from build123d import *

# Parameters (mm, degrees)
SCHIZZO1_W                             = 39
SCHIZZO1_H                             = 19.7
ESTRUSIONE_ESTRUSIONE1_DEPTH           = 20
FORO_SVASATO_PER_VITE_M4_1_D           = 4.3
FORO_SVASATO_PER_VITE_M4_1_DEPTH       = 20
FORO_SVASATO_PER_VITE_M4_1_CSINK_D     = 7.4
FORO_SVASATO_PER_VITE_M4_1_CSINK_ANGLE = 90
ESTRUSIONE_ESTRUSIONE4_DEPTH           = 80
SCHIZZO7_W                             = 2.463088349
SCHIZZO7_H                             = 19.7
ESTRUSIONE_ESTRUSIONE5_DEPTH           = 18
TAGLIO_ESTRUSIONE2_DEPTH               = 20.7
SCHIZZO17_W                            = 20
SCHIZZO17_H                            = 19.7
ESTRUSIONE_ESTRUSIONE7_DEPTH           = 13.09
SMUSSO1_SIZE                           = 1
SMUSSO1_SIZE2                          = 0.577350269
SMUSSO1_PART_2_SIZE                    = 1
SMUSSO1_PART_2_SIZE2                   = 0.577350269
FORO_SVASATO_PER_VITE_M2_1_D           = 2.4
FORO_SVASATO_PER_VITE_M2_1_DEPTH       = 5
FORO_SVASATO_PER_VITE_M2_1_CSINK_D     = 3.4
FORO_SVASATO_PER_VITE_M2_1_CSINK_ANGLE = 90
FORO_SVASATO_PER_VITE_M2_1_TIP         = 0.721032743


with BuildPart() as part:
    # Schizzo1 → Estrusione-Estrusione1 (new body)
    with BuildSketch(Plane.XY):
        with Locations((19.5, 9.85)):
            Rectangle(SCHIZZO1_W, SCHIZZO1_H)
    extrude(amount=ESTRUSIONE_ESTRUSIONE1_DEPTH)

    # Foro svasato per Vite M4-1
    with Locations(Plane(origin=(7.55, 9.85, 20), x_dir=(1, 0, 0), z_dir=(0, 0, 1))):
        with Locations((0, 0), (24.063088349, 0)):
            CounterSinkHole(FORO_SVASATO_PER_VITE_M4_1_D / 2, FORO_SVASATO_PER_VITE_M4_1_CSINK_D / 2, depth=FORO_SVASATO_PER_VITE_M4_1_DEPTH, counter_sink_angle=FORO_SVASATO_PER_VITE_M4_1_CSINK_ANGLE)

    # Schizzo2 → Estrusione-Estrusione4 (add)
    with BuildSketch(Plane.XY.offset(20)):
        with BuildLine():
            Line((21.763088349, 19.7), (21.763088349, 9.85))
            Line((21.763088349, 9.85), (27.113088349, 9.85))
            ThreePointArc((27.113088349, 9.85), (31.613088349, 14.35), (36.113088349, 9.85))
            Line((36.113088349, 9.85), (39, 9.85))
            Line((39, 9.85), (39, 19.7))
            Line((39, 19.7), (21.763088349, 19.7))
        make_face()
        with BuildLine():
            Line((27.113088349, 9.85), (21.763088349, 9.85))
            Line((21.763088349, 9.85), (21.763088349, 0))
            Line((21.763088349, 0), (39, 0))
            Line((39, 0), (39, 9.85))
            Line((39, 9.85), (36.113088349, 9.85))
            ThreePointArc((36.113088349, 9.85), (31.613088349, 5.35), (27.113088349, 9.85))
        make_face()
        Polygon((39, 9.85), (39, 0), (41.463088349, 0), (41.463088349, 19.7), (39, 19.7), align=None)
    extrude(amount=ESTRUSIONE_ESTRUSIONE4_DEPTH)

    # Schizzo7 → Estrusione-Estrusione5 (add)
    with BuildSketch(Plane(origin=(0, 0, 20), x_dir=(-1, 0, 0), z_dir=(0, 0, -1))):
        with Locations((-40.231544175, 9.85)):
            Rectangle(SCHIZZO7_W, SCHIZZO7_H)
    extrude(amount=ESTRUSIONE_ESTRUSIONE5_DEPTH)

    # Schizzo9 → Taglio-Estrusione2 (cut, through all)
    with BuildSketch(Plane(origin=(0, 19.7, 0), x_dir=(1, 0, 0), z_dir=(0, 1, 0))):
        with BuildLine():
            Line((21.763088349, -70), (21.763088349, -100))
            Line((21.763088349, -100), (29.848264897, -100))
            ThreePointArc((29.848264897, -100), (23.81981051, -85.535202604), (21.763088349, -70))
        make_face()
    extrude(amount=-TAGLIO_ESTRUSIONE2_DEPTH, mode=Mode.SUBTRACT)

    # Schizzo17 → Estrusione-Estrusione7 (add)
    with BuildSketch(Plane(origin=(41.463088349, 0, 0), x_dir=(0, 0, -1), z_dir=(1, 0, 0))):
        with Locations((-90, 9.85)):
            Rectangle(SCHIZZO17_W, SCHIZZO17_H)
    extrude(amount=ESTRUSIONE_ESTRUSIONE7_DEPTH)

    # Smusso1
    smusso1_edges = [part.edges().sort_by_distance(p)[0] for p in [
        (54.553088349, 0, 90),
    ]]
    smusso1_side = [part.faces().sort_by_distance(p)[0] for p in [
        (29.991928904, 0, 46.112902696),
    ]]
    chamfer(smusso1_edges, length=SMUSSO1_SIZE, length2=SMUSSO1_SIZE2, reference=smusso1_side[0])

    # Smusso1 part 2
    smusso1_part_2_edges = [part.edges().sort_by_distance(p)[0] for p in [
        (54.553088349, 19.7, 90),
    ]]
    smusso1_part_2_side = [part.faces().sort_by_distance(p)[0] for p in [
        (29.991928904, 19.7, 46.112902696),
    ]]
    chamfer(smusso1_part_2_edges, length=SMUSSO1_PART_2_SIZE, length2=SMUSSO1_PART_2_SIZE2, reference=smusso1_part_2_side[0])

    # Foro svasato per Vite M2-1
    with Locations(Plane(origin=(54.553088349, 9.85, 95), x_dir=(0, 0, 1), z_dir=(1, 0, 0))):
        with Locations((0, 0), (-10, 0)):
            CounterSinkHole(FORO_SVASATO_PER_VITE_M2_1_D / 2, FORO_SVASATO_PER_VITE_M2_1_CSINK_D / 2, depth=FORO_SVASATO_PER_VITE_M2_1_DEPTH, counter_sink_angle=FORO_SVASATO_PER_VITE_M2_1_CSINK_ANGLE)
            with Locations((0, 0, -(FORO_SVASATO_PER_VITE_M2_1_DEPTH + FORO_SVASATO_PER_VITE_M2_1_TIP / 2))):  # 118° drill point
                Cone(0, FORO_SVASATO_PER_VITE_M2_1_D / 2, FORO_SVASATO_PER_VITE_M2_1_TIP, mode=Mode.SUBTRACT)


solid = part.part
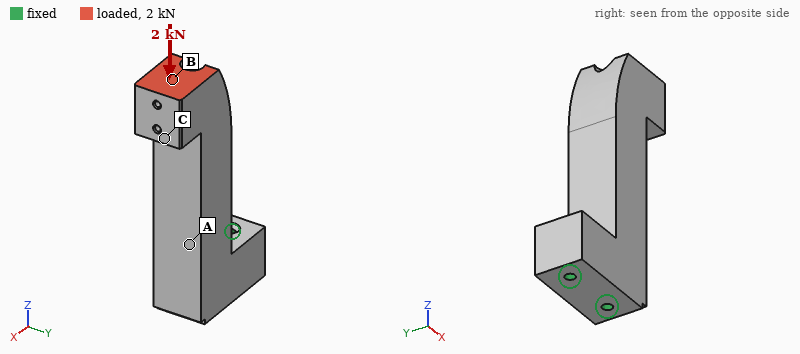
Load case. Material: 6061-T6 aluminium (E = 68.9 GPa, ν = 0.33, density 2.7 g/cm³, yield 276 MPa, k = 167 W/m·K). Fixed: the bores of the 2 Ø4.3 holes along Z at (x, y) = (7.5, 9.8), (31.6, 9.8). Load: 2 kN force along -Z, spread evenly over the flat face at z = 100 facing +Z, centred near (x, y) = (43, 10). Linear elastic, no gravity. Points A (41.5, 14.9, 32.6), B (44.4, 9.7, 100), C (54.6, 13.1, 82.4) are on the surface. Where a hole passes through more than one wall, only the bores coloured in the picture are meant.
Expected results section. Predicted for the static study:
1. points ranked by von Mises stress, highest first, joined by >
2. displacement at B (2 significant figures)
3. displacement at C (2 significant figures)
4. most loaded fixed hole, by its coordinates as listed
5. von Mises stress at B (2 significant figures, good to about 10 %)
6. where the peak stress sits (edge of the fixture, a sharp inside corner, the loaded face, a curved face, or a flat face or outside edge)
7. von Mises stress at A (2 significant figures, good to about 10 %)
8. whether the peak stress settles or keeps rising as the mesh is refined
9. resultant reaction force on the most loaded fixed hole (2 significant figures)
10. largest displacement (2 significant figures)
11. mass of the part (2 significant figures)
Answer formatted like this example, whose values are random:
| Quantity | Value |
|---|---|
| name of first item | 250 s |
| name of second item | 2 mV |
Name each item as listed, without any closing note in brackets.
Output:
| Quantity | Value |
|---|---|
| points ranked by von Mises stress, highest first, joined by > | A > B > C |
| displacement at B | 0.12 mm |
| displacement at C | 0.097 mm |
| most loaded fixed hole, by its coordinates as listed | (31.6, 9.8) |
| von Mises stress at B | 6.2 MPa |
| where the peak stress sits | edge of the fixture |
| von Mises stress at A | 25 MPa |
| whether the peak stress settles or keeps rising as the mesh is refined | keeps rising |
| resultant reaction force on the most loaded fixed hole | 2.4 kN |
| largest displacement | 0.13 mm |
| mass of the part | 120 g |
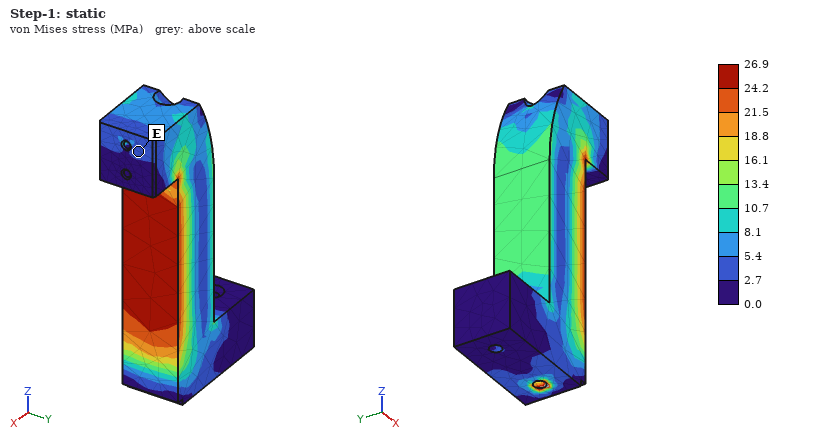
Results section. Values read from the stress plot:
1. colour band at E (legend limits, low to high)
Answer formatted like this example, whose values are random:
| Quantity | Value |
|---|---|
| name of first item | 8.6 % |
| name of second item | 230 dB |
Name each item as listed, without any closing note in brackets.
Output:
| Quantity | Value |
|---|---|
| colour band at E | 2.7 to 5.4 MPa |
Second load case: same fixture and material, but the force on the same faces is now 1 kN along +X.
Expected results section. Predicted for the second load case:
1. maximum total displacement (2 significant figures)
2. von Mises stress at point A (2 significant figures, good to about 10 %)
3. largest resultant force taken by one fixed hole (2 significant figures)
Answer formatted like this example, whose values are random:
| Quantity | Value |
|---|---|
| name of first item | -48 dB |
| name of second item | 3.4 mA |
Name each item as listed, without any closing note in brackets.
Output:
| Quantity | Value |
|---|---|
| maximum total displacement | 0.33 mm |
| von Mises stress at point A | 55 MPa |
| largest resultant force taken by one fixed hole | 2.5 kN |
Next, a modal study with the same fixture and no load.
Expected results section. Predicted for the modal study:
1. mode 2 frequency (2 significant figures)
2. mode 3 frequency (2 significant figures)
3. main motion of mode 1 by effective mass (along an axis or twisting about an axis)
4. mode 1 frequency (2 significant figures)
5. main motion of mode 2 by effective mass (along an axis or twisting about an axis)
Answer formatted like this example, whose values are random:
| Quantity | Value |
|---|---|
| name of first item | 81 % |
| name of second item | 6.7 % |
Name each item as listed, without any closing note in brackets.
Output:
| Quantity | Value |
|---|---|
| mode 2 frequency | 1800 Hz |
| mode 3 frequency | 6000 Hz |
| main motion of mode 1 by effective mass | along Y |
| mode 1 frequency | 1700 Hz |
| main motion of mode 2 by effective mass | along X |
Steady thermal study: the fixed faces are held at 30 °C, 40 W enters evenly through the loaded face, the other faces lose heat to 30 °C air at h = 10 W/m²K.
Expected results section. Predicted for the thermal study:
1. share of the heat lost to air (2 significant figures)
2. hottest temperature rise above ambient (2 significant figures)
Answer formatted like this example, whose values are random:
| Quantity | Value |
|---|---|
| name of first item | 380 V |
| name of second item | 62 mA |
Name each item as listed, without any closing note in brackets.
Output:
| Quantity | Value |
|---|---|
| share of the heat lost to air | 7.9 % |
| hottest temperature rise above ambient | 62 K |
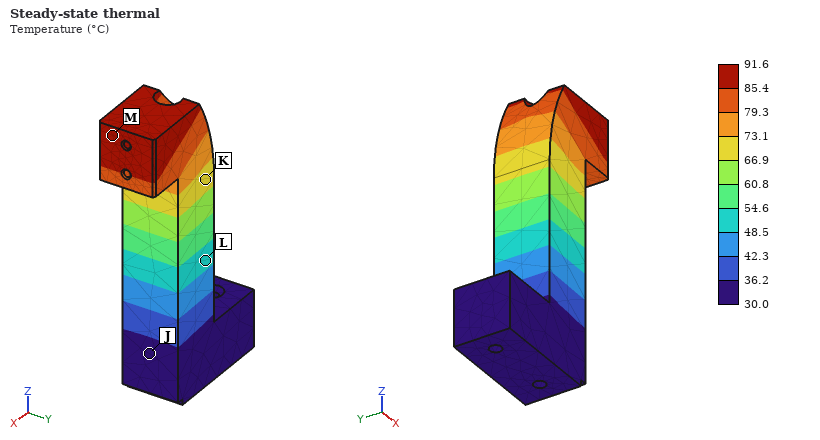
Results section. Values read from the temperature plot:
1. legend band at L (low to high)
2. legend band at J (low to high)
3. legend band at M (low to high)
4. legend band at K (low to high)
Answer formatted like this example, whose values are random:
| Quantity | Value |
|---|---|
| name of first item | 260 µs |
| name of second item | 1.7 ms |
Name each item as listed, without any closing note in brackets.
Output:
| Quantity | Value |
|---|---|
| legend band at L | 48.5 to 54.6 °C |
| legend band at J | 30.0 to 36.2 °C |
| legend band at M | 85.4 to 91.6 °C |
| legend band at K | 66.9 to 73.1 °C |
